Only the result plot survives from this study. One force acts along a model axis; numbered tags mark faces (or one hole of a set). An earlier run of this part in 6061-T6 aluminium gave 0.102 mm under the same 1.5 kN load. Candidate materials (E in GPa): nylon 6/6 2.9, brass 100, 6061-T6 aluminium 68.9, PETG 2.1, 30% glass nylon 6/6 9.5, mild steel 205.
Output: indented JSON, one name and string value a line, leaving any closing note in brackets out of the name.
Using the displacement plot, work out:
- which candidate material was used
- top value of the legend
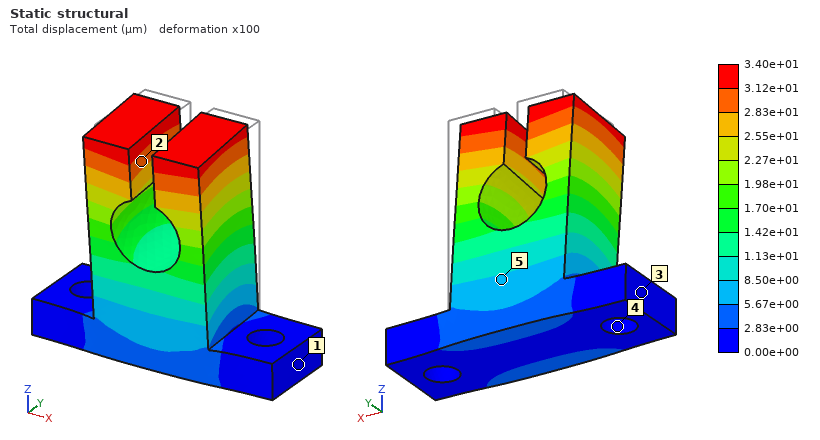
{
  "which candidate material was used": "mild steel",
  "top value of the legend": "3.40e+01 µm"
}
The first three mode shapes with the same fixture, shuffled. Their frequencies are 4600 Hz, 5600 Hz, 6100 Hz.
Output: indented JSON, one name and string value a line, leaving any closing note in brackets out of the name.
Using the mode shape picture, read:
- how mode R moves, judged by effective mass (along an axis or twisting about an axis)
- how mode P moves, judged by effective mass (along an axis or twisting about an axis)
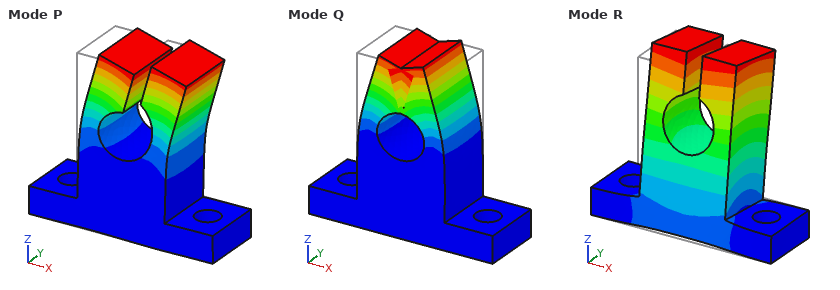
{
  "how mode R moves, judged by effective mass": "along Y",
  "how mode P moves, judged by effective mass": "along X"
}
